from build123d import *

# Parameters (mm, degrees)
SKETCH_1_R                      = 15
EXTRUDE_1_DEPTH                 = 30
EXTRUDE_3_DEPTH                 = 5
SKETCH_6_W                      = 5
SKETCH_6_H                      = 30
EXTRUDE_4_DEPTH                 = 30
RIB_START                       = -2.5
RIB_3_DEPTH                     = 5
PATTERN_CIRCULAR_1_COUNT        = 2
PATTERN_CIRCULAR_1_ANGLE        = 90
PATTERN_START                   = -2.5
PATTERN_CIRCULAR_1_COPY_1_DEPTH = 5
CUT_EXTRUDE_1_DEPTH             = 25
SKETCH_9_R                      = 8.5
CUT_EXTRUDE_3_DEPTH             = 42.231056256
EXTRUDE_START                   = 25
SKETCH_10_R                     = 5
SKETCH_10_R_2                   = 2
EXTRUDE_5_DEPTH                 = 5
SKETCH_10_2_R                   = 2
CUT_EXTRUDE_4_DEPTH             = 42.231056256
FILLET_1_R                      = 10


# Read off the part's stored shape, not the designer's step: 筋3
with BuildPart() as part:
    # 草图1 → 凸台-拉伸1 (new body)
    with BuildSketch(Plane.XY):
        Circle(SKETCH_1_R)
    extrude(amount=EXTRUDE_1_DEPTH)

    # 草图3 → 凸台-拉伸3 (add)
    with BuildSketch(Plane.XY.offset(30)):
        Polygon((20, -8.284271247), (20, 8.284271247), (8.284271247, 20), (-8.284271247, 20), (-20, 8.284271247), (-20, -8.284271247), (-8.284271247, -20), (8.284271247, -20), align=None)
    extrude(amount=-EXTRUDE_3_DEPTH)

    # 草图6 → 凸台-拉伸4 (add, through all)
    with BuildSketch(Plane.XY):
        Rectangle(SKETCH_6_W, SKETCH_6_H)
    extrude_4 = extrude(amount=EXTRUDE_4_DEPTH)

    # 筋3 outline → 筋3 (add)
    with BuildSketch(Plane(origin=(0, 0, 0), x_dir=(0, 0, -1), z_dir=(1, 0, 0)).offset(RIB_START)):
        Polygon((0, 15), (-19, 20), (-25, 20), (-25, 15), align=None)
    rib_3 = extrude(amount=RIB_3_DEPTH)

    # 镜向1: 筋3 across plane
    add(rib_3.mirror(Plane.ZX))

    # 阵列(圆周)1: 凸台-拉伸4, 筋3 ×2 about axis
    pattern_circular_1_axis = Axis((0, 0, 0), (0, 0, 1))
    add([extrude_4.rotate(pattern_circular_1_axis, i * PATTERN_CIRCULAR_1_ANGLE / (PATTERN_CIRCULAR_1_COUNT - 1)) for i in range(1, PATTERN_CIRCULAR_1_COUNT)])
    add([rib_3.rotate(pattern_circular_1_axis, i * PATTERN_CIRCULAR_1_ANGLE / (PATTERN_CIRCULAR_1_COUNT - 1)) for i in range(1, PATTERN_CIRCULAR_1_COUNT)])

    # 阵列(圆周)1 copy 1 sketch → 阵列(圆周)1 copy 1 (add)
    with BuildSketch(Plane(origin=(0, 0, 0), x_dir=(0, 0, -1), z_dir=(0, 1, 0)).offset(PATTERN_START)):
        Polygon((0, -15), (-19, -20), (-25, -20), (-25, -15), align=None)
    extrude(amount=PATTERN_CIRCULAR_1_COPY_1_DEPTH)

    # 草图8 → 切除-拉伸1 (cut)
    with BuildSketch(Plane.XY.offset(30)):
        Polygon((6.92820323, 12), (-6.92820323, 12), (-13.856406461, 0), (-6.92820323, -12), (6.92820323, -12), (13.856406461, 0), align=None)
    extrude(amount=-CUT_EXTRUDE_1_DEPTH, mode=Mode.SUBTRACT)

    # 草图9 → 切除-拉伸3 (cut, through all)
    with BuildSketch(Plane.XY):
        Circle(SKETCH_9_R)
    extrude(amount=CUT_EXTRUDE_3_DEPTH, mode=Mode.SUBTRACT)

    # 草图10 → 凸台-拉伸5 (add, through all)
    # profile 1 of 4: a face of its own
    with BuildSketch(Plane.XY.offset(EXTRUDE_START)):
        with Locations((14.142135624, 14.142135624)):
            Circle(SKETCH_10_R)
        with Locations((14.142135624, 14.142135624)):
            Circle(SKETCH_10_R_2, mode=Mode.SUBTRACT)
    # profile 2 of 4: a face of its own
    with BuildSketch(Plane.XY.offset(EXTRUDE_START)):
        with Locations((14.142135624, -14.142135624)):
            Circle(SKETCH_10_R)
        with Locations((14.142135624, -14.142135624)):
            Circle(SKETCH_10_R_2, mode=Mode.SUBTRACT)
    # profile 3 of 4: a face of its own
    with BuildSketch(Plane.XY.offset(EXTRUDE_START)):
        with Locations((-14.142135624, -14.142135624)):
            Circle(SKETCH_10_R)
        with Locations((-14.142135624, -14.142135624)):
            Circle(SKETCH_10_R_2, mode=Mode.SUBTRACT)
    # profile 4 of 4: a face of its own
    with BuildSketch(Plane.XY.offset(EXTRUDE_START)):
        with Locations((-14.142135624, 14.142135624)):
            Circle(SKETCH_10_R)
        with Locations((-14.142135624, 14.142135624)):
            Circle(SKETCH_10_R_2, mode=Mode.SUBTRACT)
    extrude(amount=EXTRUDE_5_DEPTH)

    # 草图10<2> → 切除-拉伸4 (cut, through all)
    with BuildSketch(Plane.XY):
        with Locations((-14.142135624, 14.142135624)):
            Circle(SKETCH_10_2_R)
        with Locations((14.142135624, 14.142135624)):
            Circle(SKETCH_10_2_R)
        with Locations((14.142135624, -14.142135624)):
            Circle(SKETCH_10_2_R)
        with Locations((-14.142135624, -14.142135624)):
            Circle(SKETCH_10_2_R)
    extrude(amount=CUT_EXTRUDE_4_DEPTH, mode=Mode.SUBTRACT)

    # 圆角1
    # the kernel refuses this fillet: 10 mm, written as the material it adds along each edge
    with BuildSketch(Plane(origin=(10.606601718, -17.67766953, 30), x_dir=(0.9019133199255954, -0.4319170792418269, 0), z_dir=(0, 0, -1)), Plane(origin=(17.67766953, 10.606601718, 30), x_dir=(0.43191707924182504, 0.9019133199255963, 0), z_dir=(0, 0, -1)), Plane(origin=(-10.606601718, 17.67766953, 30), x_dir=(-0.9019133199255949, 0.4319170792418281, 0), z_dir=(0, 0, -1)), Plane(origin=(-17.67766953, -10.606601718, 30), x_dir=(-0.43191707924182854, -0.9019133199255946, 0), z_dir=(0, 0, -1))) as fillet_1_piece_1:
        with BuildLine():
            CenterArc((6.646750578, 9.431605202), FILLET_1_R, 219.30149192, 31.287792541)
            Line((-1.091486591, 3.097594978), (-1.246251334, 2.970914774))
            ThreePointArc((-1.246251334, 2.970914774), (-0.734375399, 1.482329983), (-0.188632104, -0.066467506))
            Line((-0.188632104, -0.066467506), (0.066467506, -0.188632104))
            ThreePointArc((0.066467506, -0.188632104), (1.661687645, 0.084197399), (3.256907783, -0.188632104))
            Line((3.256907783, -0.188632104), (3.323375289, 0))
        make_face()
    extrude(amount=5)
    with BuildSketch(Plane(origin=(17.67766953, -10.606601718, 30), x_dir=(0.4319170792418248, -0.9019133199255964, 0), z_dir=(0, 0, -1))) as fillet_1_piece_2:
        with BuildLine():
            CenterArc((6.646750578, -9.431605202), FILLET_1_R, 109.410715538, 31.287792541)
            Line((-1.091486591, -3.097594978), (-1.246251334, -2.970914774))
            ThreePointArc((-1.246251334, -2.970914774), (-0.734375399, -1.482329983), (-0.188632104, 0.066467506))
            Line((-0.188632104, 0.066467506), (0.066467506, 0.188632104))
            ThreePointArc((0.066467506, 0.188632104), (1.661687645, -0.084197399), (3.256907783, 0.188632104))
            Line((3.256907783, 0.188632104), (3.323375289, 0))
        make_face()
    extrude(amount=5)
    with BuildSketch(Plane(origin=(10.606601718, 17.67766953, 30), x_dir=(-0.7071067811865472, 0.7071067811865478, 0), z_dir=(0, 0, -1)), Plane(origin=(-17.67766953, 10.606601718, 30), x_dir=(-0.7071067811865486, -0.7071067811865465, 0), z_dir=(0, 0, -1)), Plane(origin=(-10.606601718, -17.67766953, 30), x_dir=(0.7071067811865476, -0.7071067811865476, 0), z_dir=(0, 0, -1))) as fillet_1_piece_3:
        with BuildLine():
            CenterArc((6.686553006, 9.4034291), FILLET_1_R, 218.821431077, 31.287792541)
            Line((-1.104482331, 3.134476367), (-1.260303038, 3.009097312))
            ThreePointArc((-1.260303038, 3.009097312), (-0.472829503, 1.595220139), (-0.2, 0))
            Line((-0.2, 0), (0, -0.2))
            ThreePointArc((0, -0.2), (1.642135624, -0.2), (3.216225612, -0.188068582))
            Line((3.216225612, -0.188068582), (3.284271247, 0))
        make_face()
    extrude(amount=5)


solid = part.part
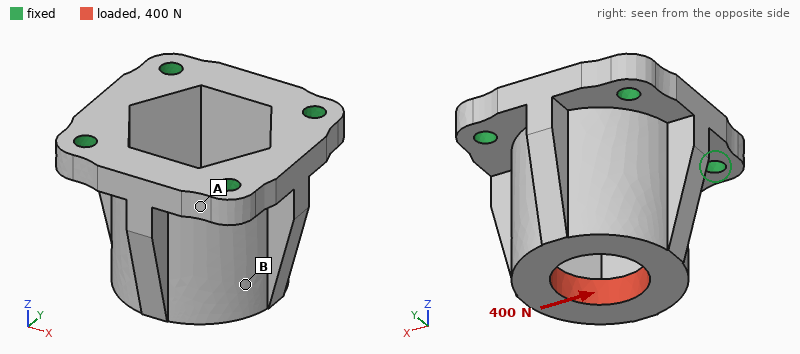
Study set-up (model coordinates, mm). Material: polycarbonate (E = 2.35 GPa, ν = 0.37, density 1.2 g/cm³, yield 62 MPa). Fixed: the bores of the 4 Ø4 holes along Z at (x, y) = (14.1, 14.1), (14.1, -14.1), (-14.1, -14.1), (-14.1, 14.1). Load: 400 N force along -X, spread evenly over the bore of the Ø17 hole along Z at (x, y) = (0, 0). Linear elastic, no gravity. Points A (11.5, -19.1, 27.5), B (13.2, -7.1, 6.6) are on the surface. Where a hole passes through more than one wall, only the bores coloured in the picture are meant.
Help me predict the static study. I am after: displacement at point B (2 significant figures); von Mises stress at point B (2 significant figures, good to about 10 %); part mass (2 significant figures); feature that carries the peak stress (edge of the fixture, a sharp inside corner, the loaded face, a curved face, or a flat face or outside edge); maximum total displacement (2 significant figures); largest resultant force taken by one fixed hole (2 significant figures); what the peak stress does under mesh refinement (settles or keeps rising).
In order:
0.20 mm
3.2 MPa
16 g
edge of the fixture
0.25 mm
210 N
keeps rising
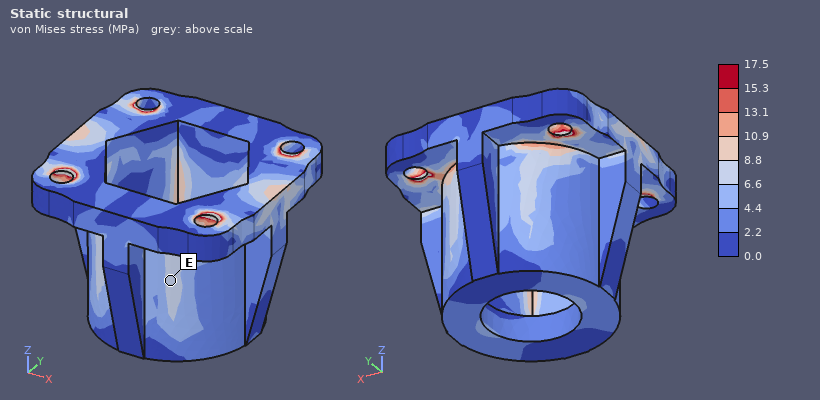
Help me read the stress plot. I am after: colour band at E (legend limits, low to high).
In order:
6.6 to 8.8 MPa
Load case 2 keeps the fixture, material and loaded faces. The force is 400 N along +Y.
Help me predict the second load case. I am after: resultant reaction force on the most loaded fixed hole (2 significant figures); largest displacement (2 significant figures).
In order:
220 N
0.24 mm
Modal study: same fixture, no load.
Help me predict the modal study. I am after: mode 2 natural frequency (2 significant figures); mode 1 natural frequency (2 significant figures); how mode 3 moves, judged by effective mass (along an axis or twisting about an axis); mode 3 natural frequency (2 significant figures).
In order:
3000 Hz
2900 Hz
along Z
5300 Hz
